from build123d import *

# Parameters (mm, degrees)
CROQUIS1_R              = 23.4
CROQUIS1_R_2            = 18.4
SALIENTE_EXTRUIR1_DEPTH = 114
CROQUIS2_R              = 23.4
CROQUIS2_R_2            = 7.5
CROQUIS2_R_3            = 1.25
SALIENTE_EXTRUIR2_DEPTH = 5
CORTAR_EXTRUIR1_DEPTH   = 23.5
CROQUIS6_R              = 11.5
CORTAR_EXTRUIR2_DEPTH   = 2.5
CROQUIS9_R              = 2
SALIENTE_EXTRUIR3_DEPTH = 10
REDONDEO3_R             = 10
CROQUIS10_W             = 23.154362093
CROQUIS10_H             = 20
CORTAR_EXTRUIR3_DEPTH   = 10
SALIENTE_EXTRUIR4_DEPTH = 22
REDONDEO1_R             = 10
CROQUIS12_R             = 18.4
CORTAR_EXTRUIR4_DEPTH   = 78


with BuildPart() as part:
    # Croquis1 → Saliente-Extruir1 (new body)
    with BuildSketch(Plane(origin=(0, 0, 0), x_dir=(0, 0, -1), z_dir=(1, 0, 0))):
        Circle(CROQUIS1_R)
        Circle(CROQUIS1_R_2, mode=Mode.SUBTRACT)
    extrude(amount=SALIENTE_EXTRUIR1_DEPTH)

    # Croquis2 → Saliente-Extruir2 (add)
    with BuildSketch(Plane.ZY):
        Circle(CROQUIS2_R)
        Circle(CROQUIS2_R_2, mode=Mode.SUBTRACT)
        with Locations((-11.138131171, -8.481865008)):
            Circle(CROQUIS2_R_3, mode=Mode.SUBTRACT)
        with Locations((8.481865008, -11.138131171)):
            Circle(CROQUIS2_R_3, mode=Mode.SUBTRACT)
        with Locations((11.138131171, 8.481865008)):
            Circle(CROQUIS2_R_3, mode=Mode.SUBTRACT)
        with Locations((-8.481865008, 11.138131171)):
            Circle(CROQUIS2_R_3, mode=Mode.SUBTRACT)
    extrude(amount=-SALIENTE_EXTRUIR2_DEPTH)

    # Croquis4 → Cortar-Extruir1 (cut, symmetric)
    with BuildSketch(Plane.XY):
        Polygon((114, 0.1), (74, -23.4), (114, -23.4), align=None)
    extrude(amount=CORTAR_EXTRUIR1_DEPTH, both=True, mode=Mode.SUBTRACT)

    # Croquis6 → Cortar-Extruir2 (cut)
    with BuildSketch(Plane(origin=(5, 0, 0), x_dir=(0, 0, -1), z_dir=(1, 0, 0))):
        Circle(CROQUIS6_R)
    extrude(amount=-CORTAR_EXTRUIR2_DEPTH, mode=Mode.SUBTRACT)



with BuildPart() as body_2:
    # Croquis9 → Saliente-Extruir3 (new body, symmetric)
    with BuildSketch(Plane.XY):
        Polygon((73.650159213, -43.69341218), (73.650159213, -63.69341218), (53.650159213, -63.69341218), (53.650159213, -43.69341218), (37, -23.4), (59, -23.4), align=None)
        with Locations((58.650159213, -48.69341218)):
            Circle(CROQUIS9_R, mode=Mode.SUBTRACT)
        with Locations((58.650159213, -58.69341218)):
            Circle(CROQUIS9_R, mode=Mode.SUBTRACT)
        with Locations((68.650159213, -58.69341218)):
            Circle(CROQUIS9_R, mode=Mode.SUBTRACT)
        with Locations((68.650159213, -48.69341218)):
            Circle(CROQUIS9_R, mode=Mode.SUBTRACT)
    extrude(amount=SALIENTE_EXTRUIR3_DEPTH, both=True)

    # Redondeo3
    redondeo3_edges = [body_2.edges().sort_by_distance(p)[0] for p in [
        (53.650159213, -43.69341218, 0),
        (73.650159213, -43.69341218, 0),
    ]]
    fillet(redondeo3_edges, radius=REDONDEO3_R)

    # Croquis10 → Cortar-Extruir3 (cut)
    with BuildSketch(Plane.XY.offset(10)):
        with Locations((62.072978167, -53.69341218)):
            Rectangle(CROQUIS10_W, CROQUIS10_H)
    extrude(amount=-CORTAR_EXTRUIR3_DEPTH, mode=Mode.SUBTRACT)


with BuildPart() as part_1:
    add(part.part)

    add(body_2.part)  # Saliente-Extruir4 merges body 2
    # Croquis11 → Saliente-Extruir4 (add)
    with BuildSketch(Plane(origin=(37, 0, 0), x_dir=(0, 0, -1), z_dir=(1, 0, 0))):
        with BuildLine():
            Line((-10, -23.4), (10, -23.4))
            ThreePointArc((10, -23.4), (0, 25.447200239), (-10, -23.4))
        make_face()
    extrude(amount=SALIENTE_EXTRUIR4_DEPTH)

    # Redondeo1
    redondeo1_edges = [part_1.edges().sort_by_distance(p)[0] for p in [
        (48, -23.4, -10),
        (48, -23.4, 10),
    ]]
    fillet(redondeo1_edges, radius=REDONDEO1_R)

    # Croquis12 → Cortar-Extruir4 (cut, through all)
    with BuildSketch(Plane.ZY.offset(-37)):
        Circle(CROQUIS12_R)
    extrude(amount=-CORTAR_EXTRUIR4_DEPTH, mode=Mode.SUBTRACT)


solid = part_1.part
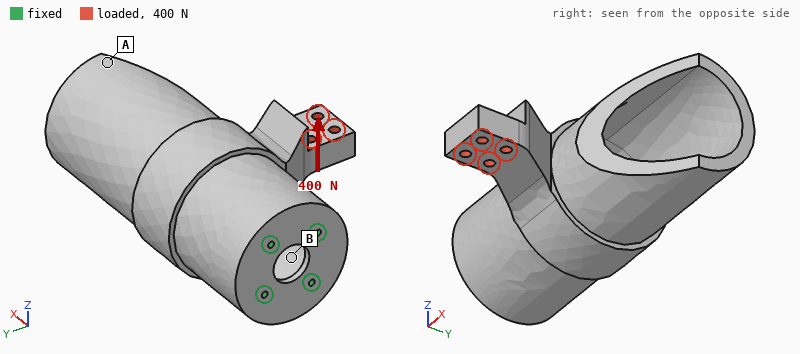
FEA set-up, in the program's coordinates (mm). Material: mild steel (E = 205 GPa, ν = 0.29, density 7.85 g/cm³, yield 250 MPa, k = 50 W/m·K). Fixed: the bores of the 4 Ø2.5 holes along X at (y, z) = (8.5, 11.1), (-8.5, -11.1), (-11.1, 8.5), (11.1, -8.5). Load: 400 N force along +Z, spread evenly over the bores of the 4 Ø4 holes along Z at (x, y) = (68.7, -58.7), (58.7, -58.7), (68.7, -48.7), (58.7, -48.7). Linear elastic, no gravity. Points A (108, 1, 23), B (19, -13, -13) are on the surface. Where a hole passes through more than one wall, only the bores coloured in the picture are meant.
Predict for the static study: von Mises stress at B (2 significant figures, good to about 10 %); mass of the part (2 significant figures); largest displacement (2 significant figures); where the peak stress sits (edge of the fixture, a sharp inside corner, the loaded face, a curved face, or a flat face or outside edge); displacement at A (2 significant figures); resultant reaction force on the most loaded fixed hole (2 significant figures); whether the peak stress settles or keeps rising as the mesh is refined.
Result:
6.3 MPa
700 g
24 µm
edge of the fixture
15 µm
730 N
keeps rising
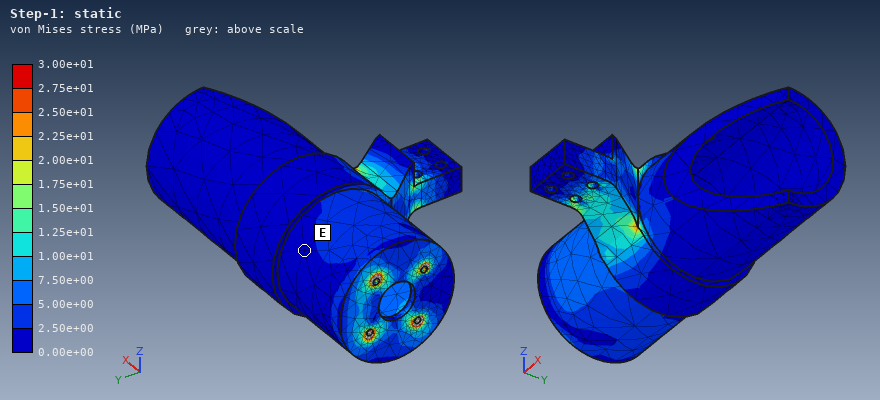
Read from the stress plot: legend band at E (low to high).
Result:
0.00e+00 to 2.50e+00 MPa
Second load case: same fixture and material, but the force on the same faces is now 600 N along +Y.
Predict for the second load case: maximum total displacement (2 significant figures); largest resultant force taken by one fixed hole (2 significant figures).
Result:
27 µm
840 N
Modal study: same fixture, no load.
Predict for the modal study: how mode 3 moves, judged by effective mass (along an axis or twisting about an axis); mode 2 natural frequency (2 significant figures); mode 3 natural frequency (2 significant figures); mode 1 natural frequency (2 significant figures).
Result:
twisting about X
1400 Hz
4500 Hz
1300 Hz
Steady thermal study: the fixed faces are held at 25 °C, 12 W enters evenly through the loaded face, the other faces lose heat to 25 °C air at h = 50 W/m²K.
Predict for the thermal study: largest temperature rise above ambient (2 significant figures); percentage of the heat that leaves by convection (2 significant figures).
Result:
38 K
76 %
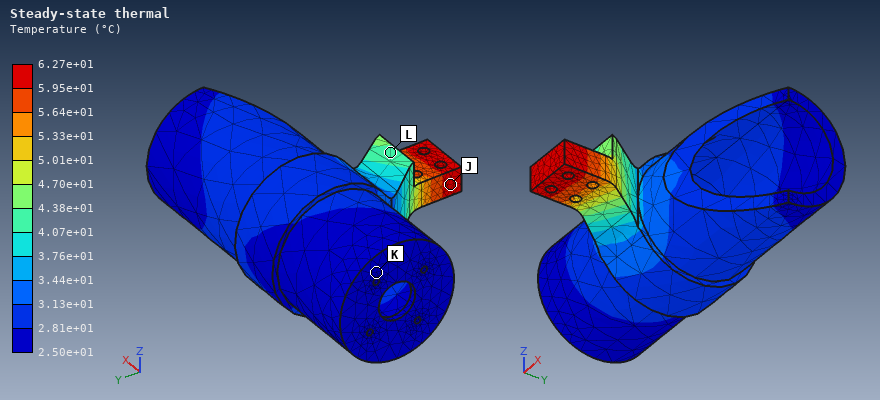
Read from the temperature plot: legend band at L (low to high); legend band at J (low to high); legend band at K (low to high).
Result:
4.07e+01 to 4.38e+01 °C
5.95e+01 to 6.27e+01 °C
2.50e+01 to 2.81e+01 °C
